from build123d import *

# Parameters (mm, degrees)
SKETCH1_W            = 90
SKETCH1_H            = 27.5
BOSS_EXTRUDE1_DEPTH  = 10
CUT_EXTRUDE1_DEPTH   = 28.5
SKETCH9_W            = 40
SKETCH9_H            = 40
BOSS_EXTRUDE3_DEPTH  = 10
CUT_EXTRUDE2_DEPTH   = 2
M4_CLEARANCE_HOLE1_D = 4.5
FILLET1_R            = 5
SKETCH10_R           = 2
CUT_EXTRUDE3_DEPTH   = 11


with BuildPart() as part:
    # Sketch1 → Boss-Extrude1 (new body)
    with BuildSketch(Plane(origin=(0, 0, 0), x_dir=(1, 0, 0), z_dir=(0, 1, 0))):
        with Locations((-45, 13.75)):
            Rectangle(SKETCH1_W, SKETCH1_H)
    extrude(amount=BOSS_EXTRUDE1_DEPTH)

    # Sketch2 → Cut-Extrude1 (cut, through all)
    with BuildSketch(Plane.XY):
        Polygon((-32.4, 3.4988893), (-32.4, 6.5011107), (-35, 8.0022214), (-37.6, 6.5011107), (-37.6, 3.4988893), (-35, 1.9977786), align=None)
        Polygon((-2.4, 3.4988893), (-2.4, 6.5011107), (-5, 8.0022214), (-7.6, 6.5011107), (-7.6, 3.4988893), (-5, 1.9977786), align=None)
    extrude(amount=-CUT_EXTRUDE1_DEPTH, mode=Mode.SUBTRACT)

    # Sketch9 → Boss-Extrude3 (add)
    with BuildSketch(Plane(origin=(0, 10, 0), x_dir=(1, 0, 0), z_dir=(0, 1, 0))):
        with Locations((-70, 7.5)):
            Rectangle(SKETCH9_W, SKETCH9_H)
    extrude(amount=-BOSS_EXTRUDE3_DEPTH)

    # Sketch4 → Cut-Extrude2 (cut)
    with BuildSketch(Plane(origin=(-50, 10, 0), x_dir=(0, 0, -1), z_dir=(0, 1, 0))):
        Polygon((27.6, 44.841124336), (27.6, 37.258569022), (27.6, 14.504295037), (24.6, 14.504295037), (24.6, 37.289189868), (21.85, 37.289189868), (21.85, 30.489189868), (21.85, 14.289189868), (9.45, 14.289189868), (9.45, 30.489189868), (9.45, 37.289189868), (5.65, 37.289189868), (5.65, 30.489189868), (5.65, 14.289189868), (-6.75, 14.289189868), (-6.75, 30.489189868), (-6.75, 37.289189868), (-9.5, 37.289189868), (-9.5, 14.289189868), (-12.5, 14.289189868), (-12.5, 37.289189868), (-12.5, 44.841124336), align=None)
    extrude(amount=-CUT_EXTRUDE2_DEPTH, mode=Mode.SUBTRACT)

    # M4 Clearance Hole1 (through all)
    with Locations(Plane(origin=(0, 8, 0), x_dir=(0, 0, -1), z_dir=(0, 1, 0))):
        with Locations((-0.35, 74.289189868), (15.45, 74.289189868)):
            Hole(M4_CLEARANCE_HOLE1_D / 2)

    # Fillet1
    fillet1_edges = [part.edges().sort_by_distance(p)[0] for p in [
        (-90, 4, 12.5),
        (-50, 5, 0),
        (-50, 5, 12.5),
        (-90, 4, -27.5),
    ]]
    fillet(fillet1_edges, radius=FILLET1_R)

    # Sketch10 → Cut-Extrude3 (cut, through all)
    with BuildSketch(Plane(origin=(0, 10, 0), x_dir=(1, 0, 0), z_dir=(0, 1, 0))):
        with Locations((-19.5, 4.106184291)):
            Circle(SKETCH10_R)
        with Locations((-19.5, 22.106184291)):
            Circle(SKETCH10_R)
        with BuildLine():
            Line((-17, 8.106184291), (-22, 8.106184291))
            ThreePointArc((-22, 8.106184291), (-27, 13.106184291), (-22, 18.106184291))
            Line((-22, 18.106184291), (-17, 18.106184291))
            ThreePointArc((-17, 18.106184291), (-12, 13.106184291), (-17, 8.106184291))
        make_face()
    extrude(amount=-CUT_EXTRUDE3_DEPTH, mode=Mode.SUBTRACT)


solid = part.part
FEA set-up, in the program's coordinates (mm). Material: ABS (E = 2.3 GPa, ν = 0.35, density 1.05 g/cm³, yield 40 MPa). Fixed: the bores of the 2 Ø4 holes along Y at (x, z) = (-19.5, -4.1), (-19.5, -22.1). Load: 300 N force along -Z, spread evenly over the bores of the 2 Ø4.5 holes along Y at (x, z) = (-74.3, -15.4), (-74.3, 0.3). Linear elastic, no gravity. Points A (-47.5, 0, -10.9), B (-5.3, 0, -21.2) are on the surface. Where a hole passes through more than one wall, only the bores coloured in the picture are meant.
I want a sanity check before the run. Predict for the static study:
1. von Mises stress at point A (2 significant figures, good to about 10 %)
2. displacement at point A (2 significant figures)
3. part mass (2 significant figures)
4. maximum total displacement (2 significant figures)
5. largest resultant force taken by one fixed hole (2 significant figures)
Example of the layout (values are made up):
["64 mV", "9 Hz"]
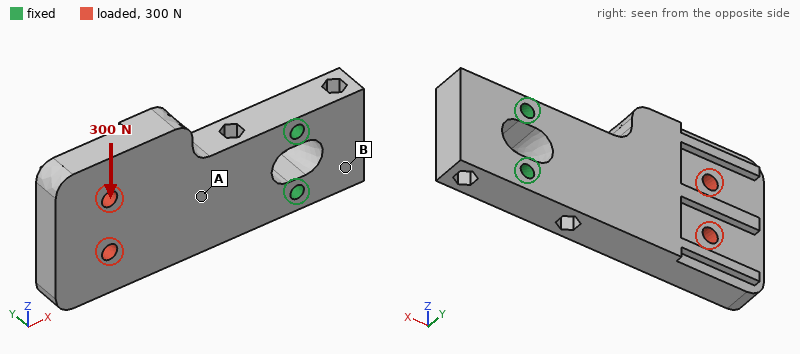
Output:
["4.1 MPa", "0.24 mm", "26 g", "0.89 mm", "820 N"]
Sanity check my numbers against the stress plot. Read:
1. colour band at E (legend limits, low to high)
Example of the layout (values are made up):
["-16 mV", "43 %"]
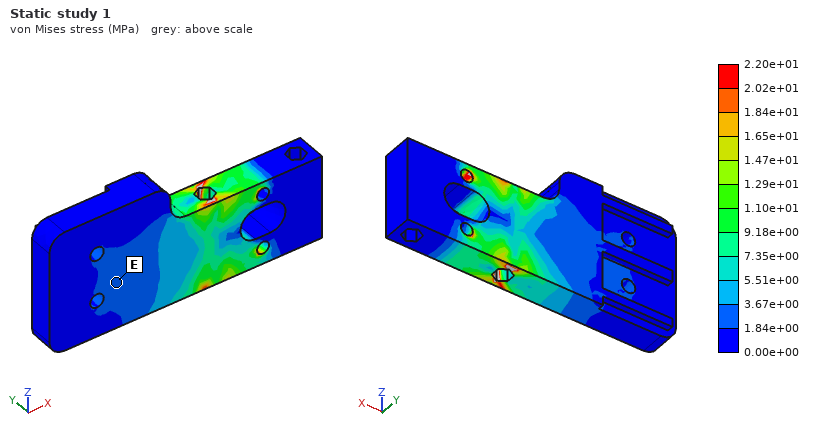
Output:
["1.84e+00 to 3.67e+00 MPa"]
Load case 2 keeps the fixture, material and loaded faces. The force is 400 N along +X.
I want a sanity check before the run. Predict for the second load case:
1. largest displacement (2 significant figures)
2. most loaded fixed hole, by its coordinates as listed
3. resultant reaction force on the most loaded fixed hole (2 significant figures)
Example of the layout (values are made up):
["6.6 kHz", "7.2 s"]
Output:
["0.27 mm", "(-19.5, -4.1)", "320 N"]
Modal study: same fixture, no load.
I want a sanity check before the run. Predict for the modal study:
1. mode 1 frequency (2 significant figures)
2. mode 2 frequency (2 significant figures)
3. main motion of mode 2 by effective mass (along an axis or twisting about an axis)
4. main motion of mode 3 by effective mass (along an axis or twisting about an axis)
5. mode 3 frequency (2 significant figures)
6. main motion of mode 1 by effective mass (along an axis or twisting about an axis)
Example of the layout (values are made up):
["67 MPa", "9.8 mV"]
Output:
["390 Hz", "940 Hz", "along Z", "twisting about X", "1300 Hz", "along Y"]
